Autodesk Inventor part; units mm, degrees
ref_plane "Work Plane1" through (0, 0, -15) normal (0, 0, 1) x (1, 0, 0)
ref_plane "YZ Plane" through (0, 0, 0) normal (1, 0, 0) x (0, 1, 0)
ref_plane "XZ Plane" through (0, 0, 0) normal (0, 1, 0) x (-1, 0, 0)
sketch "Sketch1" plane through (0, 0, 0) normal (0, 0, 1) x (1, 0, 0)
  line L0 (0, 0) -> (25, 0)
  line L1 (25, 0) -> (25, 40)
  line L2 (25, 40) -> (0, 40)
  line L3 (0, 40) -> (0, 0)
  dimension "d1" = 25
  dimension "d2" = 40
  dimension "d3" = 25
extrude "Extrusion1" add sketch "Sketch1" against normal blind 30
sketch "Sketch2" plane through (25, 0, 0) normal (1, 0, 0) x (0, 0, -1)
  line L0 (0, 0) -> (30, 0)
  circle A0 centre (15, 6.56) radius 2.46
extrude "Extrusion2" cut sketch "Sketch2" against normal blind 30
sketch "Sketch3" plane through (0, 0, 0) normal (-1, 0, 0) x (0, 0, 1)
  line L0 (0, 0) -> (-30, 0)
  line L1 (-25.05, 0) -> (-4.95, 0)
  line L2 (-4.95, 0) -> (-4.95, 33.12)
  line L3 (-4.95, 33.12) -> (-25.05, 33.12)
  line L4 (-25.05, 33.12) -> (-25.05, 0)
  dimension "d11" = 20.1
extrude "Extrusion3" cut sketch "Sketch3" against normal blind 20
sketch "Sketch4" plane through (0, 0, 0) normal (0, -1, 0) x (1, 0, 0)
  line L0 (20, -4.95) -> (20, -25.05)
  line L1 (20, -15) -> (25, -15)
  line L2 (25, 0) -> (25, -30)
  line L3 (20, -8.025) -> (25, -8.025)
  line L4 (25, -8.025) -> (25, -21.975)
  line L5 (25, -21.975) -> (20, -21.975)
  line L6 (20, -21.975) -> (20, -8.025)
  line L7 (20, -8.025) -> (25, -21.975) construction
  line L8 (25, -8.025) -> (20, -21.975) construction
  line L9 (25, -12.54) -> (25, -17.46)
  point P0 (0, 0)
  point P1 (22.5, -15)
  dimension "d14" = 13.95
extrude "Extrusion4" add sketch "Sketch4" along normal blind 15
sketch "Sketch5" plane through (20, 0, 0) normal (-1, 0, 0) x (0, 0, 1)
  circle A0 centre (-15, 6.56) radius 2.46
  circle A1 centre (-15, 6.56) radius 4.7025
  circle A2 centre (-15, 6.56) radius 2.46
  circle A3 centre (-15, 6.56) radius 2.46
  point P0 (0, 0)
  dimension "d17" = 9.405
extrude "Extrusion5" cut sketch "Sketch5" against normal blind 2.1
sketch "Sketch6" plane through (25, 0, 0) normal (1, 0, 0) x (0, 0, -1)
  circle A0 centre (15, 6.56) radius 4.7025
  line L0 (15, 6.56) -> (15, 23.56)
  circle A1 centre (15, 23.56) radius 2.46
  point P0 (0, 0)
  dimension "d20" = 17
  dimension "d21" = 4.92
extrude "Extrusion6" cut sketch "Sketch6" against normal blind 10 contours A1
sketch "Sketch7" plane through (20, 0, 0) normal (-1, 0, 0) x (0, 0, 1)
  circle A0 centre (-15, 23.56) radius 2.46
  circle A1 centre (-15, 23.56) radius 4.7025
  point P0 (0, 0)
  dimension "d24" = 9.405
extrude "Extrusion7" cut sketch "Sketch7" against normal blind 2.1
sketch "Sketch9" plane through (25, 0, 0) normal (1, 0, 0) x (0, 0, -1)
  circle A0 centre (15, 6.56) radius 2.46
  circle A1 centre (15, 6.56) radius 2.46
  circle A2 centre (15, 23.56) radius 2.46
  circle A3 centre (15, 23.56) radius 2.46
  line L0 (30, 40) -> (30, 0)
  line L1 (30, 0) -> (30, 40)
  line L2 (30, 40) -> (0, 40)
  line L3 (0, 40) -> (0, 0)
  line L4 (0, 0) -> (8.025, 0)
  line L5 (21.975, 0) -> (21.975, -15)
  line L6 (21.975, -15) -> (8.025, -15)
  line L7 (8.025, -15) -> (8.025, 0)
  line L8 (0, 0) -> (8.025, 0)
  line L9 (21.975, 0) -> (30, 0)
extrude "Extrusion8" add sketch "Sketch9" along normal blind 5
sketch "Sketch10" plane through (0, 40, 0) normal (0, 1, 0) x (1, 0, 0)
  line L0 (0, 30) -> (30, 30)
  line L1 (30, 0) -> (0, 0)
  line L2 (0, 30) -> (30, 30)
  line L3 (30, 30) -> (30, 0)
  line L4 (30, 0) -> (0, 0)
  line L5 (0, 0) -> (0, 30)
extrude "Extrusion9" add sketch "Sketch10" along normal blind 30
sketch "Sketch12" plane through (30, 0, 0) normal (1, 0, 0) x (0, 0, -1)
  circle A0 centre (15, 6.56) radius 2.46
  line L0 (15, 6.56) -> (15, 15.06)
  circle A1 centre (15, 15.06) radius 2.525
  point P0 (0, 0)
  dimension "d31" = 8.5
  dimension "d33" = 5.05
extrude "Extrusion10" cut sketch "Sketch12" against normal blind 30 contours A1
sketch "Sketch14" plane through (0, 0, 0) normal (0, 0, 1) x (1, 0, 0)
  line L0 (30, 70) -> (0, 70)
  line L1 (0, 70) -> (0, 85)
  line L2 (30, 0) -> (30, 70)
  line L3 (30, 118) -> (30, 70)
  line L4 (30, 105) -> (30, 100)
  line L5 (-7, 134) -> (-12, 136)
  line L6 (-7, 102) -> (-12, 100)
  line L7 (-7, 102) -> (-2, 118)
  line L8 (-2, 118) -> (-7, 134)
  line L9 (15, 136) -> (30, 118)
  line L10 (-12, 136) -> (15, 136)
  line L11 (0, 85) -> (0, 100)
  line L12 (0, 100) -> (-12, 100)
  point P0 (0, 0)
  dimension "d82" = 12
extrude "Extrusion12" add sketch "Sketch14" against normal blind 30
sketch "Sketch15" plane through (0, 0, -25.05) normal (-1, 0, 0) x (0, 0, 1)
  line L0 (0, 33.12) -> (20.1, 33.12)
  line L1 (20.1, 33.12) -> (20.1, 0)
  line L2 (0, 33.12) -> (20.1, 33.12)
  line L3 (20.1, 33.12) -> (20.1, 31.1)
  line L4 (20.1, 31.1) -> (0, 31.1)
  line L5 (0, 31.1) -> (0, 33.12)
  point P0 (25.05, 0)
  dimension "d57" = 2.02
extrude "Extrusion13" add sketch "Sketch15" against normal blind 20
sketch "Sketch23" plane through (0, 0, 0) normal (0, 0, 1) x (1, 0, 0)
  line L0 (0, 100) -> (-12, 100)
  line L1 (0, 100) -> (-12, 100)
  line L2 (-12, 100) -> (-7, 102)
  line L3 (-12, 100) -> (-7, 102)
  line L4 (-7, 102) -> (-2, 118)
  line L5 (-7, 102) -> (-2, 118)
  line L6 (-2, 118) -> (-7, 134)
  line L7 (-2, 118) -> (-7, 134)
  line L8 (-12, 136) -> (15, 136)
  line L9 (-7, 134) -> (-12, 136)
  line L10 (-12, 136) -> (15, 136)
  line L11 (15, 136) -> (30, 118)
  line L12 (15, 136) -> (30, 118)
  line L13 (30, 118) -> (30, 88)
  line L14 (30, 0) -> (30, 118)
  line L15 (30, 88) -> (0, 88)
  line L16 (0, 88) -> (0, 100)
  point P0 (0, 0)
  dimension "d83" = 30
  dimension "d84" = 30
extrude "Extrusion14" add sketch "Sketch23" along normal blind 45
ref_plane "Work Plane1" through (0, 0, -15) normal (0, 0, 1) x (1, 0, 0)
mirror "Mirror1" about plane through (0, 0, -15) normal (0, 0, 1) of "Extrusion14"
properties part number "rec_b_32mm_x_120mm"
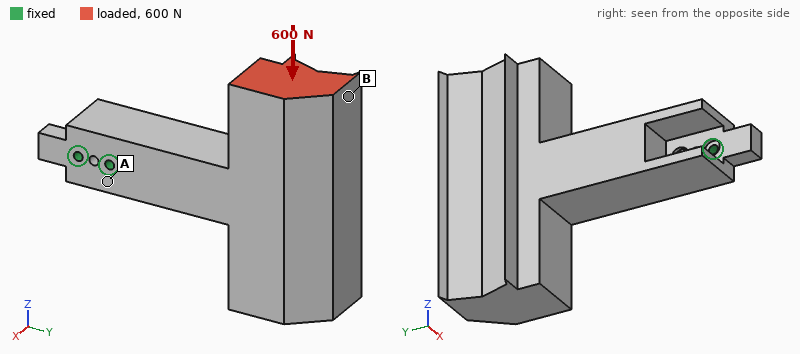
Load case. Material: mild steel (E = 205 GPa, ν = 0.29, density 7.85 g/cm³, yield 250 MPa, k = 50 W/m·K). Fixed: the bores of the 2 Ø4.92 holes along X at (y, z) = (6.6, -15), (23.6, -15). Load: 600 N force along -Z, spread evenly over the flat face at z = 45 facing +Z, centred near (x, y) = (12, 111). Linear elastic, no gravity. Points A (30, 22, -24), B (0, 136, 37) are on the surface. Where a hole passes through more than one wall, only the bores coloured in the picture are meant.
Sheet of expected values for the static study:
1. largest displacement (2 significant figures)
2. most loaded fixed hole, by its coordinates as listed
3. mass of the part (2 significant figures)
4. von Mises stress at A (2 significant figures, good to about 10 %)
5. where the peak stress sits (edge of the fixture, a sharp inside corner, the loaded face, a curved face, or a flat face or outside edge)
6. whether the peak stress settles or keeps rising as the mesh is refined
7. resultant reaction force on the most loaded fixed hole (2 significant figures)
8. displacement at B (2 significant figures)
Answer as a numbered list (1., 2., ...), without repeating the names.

1. 49 µm
2. (23.6, -15)
3. 1.9 kg
4. 17 MPa
5. edge of the fixture
6. keeps rising
7. 2.8 kN
8. 47 µm
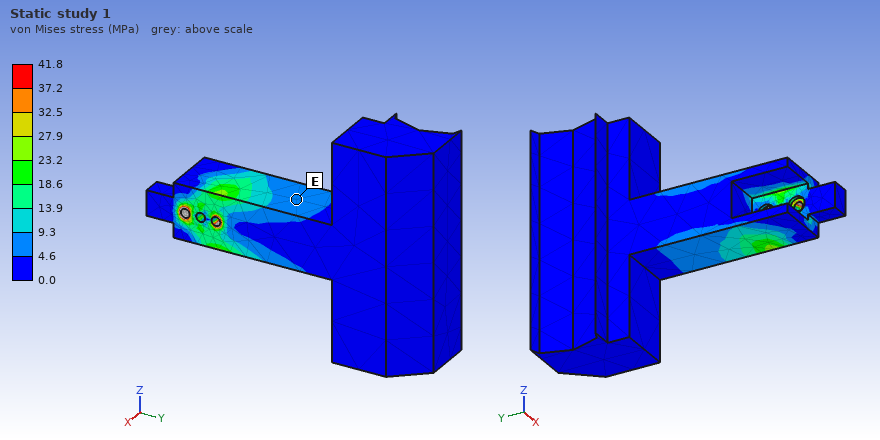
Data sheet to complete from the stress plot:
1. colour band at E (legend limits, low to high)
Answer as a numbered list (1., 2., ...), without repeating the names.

1. 4.6 to 9.3 MPa
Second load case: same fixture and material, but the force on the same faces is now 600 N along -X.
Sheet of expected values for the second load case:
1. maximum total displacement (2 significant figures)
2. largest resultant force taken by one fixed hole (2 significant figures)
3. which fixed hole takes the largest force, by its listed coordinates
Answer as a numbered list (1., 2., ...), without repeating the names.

1. 0.11 mm
2. 2.7 kN
3. (23.6, -15)
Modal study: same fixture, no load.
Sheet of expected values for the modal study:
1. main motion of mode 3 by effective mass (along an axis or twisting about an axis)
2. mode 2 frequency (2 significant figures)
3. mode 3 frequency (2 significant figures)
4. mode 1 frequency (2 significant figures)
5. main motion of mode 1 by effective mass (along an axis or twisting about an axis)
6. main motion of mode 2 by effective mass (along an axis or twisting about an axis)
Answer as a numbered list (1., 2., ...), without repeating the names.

1. twisting about Y
2. 520 Hz
3. 770 Hz
4. 480 Hz
5. along X
6. along Z
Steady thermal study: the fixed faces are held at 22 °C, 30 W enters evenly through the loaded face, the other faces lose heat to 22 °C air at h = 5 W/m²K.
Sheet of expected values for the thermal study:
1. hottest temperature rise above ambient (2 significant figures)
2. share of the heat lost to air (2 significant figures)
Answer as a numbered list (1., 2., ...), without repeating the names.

1. 73 K
2. 25 %
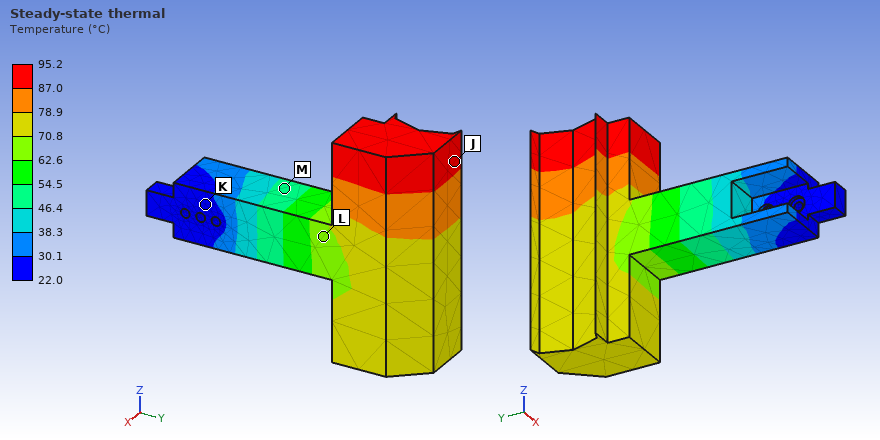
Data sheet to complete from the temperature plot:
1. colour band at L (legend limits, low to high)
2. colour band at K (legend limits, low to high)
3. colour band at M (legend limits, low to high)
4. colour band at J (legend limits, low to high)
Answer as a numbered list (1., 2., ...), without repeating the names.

1. 62.6 to 70.8 °C
2. 22.0 to 30.1 °C
3. 46.4 to 54.5 °C
4. 87.0 to 95.2 °C
